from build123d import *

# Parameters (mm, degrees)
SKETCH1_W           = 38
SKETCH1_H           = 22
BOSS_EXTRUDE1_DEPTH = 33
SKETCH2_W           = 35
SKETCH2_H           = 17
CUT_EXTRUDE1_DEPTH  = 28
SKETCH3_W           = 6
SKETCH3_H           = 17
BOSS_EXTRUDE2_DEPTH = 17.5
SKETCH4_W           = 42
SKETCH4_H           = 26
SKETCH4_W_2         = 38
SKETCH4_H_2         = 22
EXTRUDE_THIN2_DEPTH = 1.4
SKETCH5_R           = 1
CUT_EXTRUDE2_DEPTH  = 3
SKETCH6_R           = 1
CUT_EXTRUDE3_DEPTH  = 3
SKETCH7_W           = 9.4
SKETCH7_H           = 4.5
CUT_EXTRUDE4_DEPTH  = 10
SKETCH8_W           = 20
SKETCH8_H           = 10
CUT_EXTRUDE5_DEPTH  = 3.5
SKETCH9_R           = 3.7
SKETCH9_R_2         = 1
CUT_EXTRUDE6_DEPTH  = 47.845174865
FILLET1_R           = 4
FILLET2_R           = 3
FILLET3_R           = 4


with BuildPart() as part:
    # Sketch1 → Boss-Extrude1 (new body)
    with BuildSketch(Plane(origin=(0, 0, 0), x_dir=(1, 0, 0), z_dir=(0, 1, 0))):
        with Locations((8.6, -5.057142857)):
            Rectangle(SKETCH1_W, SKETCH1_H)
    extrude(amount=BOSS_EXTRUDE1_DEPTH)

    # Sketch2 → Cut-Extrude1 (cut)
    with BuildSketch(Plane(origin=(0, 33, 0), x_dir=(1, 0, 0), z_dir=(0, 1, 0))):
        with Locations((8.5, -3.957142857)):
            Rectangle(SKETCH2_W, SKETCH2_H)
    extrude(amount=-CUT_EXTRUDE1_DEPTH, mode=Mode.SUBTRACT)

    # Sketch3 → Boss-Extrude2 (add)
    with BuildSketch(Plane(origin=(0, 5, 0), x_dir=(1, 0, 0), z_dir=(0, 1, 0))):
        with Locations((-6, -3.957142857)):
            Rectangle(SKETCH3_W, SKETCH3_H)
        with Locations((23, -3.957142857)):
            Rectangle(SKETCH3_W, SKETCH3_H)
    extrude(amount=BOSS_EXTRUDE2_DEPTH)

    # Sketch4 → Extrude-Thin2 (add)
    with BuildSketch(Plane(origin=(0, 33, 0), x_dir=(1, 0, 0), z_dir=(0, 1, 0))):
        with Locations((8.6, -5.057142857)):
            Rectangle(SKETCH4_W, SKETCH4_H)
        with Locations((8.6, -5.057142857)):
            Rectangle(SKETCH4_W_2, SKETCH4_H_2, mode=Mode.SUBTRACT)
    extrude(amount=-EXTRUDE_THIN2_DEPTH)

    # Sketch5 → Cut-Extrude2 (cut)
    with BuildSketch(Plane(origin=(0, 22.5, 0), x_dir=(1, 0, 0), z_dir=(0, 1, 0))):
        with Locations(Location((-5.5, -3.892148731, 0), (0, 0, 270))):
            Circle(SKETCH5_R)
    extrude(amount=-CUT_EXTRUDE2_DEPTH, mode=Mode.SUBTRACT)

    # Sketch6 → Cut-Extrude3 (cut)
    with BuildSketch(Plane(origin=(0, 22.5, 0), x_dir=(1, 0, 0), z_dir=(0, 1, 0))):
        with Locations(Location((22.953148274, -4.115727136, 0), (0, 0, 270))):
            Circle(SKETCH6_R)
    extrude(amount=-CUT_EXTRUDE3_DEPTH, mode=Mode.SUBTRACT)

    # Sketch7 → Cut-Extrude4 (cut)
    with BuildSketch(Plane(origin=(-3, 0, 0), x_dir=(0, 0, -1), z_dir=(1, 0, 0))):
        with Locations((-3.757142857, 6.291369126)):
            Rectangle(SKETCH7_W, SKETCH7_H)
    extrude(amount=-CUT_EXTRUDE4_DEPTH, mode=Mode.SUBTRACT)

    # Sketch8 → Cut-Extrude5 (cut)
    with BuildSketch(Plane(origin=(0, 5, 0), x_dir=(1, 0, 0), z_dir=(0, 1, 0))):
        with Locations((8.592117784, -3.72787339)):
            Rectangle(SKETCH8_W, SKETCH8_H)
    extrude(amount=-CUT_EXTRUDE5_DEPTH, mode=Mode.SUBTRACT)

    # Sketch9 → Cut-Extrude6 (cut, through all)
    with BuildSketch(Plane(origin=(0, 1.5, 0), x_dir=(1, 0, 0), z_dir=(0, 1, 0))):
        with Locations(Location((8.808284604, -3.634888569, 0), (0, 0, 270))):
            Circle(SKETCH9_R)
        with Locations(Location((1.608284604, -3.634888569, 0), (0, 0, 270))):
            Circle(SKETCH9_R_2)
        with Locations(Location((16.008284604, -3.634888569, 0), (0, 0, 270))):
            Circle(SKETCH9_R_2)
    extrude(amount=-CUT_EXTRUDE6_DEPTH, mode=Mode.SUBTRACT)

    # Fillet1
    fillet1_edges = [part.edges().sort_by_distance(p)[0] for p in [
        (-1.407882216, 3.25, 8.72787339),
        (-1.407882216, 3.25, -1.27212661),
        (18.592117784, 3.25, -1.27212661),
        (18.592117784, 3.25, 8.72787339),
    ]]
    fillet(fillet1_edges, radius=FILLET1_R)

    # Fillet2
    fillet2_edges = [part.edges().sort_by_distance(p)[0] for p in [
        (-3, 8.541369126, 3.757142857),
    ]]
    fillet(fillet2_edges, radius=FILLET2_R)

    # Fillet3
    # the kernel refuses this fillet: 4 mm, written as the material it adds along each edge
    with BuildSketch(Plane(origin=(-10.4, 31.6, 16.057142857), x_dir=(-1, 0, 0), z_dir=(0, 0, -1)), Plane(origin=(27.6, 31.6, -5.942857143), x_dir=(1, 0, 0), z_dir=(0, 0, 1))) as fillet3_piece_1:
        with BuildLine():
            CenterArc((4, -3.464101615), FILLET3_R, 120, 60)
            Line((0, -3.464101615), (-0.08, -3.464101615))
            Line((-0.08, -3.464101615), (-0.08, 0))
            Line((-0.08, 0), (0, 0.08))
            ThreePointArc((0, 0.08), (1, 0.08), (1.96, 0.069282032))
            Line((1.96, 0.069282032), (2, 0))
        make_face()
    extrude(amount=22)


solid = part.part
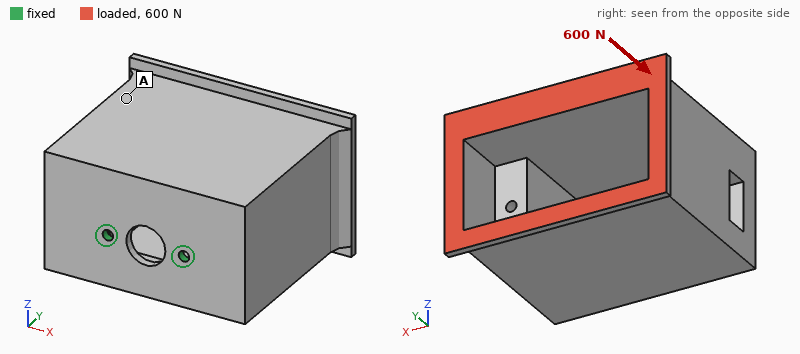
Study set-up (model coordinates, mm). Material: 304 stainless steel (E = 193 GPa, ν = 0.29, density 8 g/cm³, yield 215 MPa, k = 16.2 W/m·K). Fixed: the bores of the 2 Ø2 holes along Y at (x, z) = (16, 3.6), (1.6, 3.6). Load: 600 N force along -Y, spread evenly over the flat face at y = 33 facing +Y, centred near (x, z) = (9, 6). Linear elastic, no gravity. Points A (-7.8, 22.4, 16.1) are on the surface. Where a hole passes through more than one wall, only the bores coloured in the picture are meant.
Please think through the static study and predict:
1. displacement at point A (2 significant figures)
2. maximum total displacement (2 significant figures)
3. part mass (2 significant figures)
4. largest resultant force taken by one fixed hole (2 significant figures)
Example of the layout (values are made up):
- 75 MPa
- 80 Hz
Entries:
- 38 µm
- 53 µm
- 110 g
- 320 N
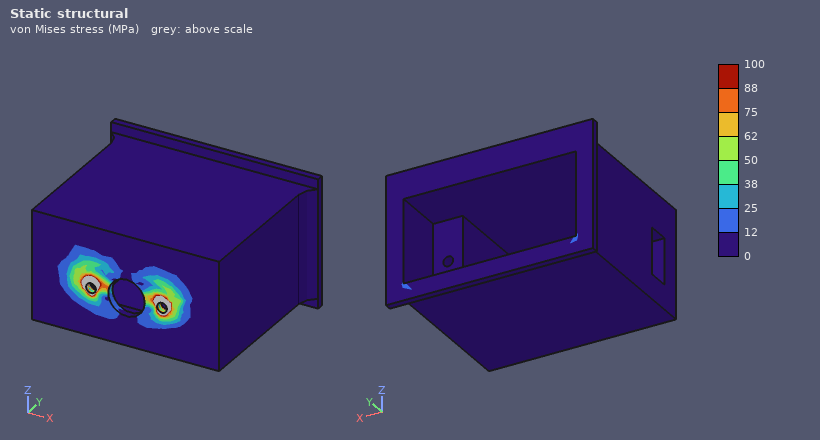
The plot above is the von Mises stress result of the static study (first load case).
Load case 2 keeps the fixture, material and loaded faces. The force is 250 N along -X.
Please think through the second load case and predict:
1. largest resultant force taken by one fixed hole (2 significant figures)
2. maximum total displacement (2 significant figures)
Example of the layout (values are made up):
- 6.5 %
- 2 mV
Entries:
- 490 N
- 26 µm
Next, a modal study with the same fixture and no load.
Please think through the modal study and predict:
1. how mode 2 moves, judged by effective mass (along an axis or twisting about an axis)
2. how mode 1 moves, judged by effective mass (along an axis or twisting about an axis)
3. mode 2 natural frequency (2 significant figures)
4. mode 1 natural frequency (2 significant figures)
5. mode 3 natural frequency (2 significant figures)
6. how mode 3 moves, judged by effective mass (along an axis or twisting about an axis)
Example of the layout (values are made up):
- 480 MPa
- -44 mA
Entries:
- along X
- along Z
- 2500 Hz
- 870 Hz
- 5600 Hz
- twisting about Y
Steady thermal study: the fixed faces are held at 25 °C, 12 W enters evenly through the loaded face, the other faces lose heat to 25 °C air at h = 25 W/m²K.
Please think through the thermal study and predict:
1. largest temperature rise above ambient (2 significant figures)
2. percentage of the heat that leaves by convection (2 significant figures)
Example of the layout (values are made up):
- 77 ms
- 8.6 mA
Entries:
- 76 K
- 70 %
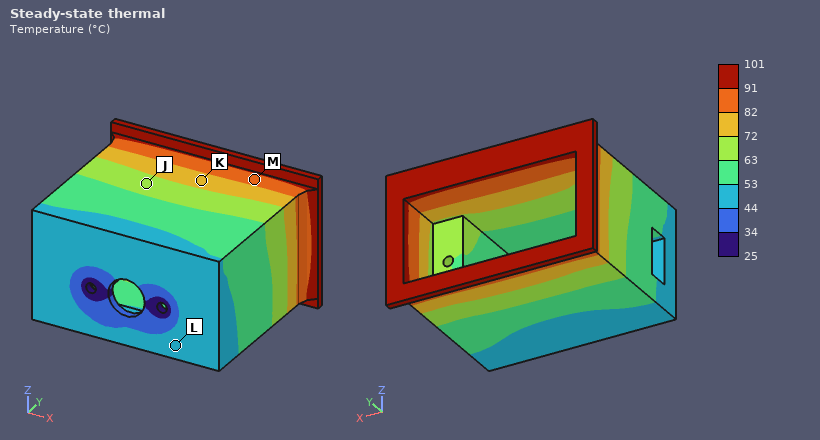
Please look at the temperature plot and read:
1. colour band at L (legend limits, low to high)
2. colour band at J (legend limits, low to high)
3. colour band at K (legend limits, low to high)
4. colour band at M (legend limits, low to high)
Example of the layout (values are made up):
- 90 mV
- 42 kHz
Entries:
- 44 to 53 °C
- 63 to 72 °C
- 72 to 82 °C
- 82 to 91 °C
